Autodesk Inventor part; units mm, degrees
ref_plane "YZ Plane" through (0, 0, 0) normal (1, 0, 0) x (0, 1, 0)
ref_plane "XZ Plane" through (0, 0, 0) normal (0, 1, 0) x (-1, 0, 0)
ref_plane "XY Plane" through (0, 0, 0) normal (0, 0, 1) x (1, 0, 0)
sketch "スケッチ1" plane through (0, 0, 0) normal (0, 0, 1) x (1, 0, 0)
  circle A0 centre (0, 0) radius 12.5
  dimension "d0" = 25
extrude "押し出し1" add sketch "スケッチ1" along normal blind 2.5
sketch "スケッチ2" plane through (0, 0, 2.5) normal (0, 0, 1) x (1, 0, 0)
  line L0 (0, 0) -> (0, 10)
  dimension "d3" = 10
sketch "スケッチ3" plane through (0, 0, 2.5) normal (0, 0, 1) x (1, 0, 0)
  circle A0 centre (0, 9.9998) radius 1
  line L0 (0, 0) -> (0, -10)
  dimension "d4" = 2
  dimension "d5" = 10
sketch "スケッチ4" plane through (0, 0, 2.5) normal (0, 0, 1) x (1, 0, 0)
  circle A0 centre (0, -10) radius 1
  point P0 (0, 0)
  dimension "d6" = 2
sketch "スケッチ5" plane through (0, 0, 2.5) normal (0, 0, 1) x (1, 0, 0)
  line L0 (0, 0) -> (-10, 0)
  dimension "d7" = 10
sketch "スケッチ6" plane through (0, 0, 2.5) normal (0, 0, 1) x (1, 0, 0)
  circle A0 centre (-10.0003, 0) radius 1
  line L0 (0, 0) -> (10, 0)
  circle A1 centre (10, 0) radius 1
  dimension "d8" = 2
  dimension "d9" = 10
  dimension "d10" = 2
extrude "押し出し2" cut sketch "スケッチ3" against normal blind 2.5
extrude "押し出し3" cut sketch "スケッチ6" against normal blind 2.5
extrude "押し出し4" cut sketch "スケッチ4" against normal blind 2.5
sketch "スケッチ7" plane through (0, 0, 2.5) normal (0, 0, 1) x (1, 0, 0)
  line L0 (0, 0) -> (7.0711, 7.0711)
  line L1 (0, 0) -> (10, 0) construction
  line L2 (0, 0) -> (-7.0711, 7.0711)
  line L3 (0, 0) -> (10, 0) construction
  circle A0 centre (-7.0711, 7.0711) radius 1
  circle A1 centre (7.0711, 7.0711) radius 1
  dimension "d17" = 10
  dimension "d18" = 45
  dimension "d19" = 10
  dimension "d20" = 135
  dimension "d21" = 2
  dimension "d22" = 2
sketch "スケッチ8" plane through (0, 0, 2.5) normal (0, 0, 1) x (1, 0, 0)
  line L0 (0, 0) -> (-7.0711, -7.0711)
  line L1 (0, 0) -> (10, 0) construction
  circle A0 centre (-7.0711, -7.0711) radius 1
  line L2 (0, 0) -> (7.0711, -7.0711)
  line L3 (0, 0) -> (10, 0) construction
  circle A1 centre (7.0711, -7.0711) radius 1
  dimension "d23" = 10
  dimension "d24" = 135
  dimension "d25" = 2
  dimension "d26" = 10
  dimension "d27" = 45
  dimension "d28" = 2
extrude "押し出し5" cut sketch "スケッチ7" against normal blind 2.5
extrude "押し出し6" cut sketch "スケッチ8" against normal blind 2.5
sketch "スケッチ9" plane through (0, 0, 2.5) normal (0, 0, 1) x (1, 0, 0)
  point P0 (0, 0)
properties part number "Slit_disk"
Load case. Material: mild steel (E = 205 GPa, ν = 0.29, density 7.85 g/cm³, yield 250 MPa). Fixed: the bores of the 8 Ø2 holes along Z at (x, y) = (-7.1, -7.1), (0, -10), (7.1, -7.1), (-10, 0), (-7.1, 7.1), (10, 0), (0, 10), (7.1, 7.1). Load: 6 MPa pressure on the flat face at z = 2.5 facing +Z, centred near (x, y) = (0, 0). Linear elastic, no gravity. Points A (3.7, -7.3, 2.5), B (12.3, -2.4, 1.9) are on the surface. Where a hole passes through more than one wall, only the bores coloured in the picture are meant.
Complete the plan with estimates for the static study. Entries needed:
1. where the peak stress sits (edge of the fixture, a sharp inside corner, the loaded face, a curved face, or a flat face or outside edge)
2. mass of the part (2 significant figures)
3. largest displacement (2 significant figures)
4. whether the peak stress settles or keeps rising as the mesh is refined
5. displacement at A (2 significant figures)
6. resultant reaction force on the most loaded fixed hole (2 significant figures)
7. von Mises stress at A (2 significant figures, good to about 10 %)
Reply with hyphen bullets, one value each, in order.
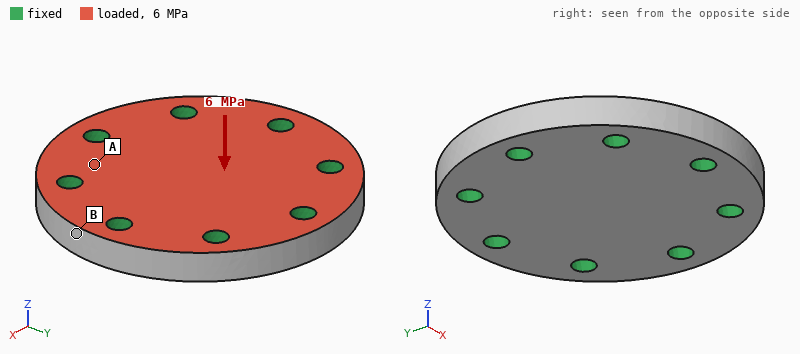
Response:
- edge of the fixture
- 9.1 g
- 3.9 µm
- keeps rising
- 0.90 µm
- 350 N
- 32 MPa
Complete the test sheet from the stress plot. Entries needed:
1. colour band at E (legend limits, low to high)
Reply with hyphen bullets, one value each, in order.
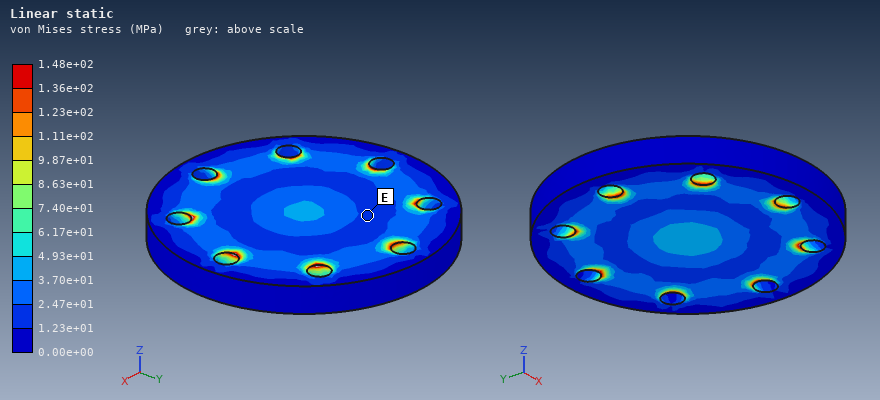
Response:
- 1.23e+01 to 2.47e+01 MPa
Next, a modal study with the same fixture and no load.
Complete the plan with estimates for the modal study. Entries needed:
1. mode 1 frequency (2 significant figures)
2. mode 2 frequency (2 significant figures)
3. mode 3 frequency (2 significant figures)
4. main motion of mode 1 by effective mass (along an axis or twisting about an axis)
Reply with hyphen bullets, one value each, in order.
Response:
- 54 kHz
- 100 kHz
- 100 kHz
- along Z
